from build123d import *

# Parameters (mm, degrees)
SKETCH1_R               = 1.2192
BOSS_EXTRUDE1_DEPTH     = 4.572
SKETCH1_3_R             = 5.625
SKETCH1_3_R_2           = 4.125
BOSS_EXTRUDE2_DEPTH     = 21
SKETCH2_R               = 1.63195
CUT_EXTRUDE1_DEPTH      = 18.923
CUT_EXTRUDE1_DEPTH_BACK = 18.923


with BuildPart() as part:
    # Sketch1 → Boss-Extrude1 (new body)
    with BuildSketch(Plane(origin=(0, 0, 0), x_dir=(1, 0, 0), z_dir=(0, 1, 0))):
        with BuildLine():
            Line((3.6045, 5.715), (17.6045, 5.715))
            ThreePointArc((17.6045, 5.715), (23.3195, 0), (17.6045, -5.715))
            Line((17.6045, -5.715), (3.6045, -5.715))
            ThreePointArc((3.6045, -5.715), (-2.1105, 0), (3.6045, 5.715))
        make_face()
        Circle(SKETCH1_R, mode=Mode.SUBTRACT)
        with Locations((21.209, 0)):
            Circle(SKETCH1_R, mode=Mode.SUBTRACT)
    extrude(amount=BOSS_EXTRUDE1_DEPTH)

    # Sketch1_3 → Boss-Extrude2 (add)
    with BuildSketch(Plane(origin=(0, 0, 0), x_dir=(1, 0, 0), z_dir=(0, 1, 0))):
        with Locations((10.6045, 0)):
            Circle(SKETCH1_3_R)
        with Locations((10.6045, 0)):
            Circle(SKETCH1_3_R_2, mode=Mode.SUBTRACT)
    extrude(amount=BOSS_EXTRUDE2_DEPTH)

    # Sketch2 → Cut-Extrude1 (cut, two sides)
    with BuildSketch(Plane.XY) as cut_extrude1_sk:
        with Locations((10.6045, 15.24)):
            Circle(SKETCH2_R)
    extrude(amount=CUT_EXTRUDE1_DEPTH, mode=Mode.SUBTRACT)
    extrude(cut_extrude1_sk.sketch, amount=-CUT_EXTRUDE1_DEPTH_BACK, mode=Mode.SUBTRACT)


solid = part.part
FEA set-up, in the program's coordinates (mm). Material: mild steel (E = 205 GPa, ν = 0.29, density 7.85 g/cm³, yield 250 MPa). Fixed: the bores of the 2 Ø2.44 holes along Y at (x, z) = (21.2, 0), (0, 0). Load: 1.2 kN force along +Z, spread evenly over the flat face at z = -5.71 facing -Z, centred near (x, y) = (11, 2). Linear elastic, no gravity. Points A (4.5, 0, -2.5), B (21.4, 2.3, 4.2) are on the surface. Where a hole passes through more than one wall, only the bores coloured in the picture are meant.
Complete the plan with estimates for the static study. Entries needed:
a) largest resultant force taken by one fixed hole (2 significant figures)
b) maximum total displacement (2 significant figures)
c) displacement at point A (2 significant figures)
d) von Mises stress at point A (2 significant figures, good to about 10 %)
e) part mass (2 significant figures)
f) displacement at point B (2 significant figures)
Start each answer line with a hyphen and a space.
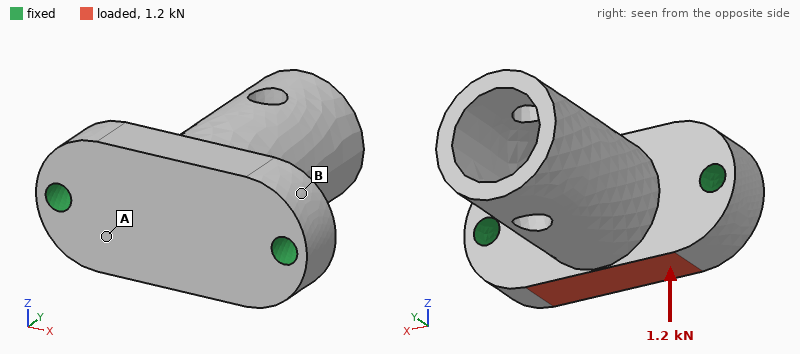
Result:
- 610 N
- 2.4 µm
- 1.3 µm
- 26 MPa
- 15 g
- 0.57 µm
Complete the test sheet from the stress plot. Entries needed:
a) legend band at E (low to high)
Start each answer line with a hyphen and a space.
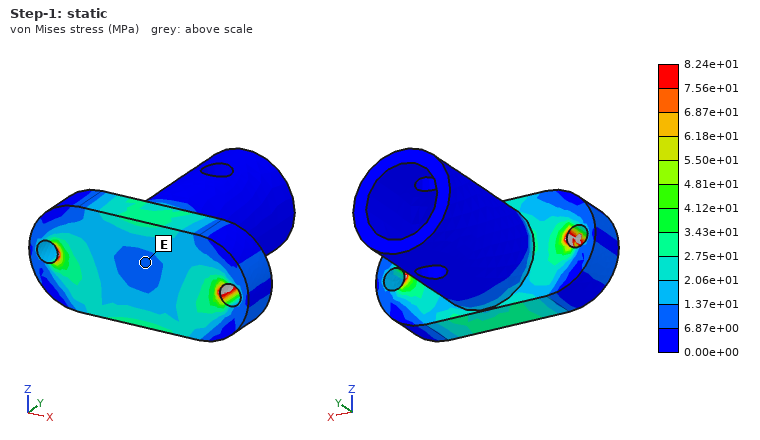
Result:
- 6.87e+00 to 1.37e+01 MPa
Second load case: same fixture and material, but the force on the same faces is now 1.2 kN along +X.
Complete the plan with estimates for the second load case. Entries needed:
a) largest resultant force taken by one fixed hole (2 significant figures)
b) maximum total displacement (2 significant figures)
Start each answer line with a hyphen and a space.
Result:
- 680 N
- 1.4 µm
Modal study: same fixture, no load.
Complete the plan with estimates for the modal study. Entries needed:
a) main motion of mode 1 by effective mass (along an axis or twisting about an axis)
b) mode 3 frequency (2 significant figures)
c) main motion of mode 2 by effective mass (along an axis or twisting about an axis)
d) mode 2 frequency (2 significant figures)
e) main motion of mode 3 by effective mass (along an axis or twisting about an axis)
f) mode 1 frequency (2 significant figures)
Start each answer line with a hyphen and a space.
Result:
- along Z
- 29 kHz
- along X
- 19 kHz
- along Y
- 11 kHz
